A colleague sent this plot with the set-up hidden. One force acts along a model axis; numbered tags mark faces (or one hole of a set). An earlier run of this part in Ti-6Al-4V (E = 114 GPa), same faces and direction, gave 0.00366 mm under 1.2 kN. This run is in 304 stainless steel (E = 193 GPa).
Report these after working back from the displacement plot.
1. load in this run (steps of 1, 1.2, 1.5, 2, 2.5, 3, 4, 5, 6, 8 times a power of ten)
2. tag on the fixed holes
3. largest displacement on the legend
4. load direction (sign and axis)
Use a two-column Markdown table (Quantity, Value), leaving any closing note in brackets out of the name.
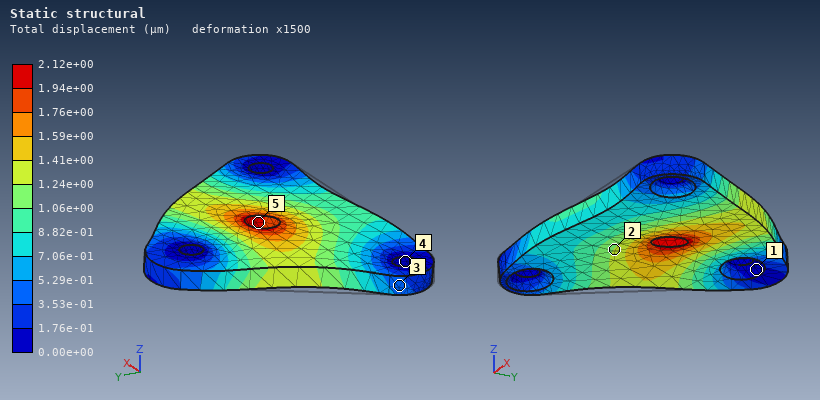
| Quantity | Value |
|---|---|
| load in this run | 1.2 kN |
| tag on the fixed holes | 4 |
| largest displacement on the legend | 2.12e+00 µm |
| load direction | +X |
